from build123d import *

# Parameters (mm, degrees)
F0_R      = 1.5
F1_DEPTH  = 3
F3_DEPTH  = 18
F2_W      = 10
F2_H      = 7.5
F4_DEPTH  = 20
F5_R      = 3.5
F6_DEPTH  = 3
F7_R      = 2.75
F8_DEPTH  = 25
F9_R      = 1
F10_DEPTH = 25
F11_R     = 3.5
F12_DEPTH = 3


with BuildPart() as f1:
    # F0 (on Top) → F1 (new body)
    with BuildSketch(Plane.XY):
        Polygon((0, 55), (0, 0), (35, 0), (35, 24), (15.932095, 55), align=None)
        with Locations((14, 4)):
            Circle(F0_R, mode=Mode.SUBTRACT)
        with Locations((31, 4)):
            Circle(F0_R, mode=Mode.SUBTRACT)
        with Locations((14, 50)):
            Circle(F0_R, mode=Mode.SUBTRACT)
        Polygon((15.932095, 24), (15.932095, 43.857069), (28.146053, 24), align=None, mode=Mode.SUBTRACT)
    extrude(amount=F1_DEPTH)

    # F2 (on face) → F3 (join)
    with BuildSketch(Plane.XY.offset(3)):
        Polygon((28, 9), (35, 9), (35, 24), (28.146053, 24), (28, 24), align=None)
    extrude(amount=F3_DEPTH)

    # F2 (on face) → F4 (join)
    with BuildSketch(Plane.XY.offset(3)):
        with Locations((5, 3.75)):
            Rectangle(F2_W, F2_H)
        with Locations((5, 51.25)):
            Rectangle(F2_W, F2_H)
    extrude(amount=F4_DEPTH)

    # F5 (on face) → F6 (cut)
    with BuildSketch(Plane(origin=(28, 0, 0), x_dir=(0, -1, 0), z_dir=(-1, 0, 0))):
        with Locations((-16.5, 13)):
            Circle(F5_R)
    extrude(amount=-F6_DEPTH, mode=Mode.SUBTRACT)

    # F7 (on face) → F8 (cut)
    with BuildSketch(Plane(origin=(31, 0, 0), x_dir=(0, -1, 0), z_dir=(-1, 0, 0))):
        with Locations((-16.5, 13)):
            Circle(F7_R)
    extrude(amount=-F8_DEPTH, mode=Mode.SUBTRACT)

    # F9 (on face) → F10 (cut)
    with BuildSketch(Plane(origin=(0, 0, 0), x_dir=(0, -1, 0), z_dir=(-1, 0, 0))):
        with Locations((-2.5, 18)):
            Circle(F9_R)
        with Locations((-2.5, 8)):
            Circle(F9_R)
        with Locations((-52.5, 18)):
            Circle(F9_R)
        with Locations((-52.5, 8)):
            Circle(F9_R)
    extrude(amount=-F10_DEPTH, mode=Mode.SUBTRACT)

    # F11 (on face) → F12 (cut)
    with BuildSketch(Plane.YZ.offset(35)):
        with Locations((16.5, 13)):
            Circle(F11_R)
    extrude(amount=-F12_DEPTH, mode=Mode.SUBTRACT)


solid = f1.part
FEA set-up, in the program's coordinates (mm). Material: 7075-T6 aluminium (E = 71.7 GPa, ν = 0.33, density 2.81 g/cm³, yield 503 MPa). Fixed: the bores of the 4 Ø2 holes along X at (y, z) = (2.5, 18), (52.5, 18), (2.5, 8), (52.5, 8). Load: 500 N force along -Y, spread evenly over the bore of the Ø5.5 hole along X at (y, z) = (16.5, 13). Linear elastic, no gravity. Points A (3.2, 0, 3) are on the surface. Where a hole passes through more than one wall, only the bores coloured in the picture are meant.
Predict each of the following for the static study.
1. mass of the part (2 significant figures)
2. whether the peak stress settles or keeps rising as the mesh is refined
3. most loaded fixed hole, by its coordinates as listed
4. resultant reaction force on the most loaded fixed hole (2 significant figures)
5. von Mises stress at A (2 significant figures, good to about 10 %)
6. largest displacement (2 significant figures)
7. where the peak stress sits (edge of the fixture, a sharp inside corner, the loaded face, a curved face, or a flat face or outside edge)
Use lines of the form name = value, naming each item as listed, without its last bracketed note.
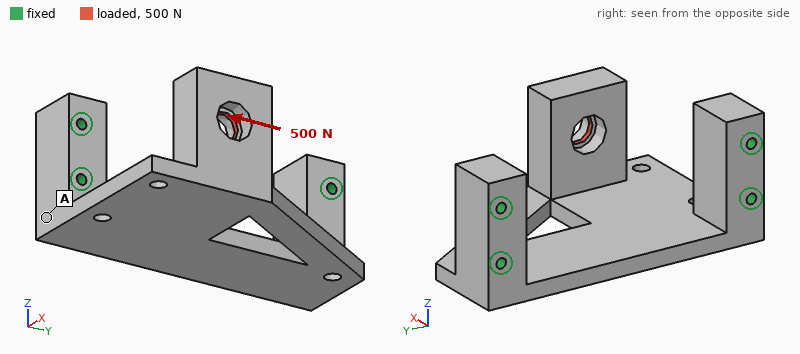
mass of the part = 25 g
whether the peak stress settles or keeps rising as the mesh is refined = keeps rising
most loaded fixed hole, by its coordinates as listed = (2.5, 8)
resultant reaction force on the most loaded fixed hole = 510 N
von Mises stress at A = 22 MPa
largest displacement = 0.27 mm
where the peak stress sits = a sharp inside corner
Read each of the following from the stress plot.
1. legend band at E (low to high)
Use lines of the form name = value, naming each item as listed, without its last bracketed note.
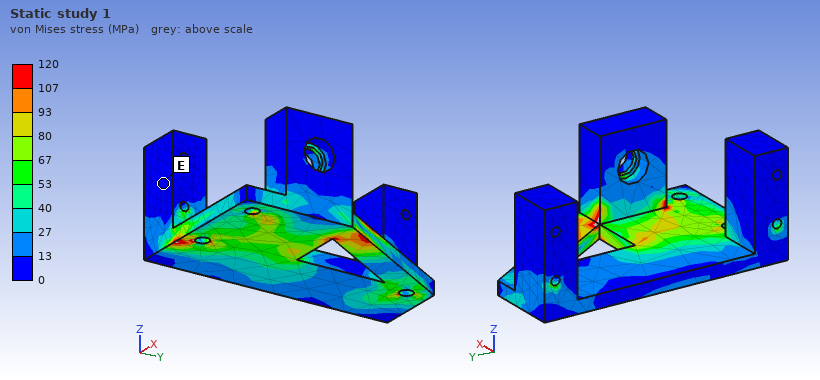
legend band at E = 0 to 13 MPa
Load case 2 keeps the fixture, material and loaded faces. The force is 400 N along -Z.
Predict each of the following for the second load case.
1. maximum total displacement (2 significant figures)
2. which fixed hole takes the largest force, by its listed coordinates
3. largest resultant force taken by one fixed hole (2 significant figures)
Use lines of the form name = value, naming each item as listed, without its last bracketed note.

maximum total displacement = 0.80 mm
which fixed hole takes the largest force, by its listed coordinates = (2.5, 8)
largest resultant force taken by one fixed hole = 250 N
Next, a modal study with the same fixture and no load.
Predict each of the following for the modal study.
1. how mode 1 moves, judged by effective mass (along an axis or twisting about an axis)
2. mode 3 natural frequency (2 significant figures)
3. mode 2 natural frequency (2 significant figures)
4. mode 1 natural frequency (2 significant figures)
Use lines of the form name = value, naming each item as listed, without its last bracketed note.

how mode 1 moves, judged by effective mass = along Z
mode 3 natural frequency = 5100 Hz
mode 2 natural frequency = 3500 Hz
mode 1 natural frequency = 1500 Hz
